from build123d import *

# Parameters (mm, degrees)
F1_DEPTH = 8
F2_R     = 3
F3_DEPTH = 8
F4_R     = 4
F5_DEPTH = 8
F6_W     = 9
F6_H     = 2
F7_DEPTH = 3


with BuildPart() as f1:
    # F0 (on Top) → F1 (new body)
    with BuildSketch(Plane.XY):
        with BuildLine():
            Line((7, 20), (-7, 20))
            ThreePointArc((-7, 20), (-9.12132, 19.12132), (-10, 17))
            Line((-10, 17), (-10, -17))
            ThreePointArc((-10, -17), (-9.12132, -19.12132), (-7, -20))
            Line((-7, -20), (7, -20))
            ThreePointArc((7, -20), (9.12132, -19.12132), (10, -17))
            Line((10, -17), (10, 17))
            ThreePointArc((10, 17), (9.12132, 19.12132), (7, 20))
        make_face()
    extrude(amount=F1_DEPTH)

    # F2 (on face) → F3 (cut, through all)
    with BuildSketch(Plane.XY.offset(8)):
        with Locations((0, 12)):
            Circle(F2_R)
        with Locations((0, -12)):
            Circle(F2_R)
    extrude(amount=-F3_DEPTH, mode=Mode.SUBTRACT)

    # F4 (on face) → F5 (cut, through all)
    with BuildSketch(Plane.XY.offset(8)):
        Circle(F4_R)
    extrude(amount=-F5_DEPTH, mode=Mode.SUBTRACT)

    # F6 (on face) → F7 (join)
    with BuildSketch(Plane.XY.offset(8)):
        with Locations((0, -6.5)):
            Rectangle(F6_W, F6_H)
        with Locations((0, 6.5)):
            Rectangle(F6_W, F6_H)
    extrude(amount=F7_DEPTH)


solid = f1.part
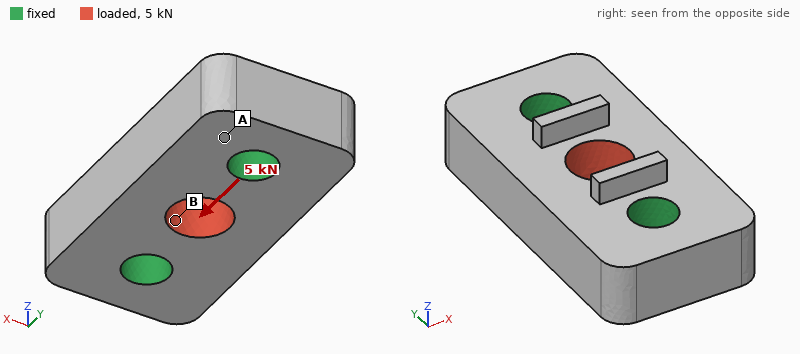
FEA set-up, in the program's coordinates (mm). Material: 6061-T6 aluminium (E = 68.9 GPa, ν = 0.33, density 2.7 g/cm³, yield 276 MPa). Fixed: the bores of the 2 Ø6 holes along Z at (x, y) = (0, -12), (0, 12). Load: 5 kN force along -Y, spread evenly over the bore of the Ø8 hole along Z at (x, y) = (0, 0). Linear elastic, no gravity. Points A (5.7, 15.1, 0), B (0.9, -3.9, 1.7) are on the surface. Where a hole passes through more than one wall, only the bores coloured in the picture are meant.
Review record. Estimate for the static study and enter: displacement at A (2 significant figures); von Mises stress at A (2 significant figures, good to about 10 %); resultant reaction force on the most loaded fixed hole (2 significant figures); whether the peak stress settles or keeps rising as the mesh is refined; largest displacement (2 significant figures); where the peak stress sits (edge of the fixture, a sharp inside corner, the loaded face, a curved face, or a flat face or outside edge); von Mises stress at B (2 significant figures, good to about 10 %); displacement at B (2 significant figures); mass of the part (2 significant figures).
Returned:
0.71 µm
6.3 MPa
2.5 kN
keeps rising
3.8 µm
edge of the fixture
31 MPa
2.4 µm
15 g
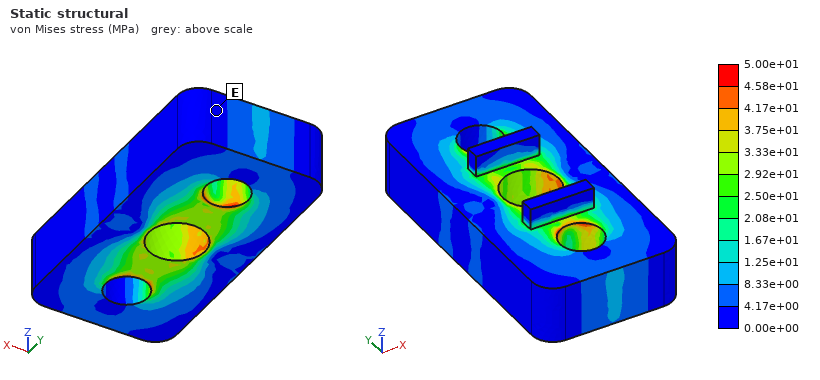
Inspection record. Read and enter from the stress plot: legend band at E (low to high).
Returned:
0.00e+00 to 4.17e+00 MPa
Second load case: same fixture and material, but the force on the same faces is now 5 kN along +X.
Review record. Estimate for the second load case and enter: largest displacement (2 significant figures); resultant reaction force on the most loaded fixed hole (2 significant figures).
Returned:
8.3 µm
2.5 kN
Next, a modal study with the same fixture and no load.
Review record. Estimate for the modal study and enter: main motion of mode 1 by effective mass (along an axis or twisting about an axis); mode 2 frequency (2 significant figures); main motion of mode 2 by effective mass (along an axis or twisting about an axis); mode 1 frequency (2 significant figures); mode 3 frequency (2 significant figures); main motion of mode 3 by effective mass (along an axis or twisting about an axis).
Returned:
twisting about Y
46 kHz
along Z
43 kHz
58 kHz
twisting about Z
